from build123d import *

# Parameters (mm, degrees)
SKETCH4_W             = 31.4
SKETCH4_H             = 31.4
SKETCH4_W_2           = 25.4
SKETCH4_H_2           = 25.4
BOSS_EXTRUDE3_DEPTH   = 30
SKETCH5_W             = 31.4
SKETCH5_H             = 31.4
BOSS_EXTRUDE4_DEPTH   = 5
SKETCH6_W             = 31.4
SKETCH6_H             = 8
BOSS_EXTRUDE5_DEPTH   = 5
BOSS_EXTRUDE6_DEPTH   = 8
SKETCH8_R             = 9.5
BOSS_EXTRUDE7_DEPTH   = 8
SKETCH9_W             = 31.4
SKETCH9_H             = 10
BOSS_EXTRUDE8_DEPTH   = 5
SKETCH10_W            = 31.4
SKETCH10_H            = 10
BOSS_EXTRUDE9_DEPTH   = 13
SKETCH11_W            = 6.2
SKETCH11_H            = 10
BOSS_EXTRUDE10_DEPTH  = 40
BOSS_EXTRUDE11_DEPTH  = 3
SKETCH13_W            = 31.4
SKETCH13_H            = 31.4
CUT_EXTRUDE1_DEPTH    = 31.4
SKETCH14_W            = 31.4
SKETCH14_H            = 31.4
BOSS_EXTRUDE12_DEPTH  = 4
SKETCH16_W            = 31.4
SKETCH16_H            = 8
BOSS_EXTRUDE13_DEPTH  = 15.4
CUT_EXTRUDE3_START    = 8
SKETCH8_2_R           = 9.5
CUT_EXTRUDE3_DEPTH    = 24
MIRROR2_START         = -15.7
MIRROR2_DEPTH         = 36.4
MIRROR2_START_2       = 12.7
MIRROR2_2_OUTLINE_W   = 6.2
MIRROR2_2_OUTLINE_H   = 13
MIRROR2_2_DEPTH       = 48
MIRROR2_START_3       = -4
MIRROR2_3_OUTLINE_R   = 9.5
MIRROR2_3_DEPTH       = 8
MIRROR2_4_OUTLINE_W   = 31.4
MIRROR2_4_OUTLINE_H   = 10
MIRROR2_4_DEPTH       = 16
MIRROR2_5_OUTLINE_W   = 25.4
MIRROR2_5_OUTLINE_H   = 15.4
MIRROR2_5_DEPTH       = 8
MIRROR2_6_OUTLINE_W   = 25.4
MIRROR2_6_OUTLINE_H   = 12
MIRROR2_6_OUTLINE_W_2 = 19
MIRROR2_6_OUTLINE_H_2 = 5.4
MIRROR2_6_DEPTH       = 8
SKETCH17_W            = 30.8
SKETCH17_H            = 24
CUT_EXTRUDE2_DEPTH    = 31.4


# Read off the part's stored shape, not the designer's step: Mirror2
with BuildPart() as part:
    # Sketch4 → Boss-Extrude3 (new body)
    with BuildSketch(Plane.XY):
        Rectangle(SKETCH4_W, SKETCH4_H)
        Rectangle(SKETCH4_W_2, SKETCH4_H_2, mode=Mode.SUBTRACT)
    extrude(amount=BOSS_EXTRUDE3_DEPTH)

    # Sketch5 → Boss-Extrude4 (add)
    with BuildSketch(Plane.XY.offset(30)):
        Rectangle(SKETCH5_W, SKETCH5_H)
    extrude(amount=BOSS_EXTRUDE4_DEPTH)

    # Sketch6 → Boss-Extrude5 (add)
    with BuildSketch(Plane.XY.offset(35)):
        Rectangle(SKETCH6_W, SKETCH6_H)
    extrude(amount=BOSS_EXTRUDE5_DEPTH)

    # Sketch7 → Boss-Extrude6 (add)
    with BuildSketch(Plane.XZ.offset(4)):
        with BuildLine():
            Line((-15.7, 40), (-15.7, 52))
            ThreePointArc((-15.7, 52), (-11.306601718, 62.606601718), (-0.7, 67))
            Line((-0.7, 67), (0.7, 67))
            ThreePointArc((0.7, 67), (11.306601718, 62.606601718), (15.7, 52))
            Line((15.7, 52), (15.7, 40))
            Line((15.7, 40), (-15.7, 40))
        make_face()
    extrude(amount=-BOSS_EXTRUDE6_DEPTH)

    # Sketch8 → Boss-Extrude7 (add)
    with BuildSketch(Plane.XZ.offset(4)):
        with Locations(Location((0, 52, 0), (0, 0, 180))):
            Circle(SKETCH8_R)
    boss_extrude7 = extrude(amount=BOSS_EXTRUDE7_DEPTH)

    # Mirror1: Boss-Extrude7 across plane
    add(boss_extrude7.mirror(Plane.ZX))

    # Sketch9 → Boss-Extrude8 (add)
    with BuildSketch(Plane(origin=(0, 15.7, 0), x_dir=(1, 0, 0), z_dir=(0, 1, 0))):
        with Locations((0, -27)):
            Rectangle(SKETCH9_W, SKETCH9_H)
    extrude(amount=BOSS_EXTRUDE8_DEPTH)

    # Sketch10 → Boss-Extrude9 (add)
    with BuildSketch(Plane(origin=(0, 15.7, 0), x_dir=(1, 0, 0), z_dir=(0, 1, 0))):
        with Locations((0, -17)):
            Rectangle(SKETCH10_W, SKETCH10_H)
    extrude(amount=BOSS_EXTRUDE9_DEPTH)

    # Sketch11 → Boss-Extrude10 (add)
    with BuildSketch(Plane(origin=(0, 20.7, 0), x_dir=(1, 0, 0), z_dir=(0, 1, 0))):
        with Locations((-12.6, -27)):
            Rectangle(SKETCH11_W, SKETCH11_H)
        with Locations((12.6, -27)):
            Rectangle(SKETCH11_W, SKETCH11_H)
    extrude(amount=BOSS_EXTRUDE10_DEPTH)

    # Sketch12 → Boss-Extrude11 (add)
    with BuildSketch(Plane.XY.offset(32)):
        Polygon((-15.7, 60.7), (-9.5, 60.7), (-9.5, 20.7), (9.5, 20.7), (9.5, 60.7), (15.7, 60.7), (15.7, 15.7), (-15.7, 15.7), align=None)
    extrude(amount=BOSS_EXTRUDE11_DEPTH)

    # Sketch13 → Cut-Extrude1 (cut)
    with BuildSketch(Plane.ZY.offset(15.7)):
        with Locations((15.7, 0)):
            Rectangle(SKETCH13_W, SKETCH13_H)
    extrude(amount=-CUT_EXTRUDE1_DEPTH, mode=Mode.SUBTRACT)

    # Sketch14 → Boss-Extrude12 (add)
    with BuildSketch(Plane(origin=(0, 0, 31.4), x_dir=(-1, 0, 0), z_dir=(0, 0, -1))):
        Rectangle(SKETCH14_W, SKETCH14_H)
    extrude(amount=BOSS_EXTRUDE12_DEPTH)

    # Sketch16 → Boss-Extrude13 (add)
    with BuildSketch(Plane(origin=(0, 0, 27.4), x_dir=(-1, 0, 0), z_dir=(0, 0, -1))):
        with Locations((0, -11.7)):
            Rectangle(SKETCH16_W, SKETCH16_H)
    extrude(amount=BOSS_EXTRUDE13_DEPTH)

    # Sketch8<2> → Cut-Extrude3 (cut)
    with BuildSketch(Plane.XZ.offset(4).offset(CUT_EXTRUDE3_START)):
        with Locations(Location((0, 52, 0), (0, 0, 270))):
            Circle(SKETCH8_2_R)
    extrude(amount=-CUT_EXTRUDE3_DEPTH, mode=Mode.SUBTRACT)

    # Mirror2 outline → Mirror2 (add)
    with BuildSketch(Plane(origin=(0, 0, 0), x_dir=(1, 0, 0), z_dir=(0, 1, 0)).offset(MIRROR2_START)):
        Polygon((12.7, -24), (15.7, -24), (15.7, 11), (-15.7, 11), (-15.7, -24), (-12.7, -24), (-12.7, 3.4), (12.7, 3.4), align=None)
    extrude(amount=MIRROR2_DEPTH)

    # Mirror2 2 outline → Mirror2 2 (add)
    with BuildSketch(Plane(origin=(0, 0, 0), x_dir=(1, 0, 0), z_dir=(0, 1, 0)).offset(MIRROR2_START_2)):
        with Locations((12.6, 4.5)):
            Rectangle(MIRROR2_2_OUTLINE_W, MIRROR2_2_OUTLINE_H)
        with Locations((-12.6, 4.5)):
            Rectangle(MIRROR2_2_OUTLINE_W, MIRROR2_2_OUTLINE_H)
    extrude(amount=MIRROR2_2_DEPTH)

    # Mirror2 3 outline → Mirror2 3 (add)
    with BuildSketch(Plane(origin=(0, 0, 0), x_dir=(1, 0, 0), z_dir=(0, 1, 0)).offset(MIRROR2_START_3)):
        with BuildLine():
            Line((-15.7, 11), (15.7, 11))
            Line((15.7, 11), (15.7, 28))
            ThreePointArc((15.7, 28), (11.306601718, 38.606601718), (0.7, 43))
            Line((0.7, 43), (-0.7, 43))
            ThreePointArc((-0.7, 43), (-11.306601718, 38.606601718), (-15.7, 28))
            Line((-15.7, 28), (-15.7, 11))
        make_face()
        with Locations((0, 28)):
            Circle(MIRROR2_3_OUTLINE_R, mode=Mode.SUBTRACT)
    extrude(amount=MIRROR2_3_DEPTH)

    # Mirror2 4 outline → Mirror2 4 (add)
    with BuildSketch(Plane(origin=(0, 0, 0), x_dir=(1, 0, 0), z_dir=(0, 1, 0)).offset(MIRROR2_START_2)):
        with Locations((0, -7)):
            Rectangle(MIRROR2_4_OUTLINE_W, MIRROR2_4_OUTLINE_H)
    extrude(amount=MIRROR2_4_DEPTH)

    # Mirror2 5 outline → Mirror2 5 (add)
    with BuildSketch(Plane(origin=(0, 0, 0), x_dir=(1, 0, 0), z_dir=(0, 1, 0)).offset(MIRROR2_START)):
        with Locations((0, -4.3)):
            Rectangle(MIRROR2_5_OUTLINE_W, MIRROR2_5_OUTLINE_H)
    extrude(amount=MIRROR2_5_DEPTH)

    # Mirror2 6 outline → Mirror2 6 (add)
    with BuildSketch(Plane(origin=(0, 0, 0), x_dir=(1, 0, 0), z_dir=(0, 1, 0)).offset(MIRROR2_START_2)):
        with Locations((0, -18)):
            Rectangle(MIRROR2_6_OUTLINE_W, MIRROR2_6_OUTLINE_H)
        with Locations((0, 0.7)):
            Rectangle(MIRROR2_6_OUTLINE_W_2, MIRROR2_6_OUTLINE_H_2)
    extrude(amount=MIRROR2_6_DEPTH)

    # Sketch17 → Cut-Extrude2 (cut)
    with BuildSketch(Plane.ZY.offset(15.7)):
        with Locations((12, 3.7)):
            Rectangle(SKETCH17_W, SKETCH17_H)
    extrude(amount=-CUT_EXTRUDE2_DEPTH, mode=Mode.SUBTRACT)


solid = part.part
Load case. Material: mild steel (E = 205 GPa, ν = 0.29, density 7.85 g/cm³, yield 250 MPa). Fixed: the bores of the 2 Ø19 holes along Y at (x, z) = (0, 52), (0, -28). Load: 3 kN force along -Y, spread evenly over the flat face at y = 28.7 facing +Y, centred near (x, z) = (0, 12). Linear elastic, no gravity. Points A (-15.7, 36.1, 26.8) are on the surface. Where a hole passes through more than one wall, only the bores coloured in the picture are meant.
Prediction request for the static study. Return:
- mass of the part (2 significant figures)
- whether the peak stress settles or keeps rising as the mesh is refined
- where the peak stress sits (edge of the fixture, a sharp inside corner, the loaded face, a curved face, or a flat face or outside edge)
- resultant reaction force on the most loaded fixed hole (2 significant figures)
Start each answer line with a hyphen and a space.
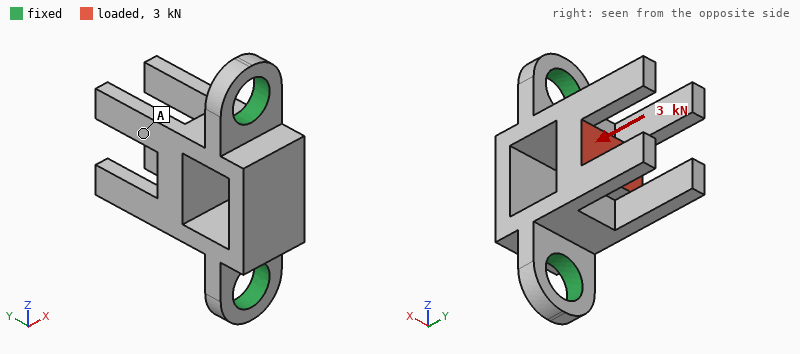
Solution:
- 450 g
- keeps rising
- edge of the fixture
- 1.6 kN
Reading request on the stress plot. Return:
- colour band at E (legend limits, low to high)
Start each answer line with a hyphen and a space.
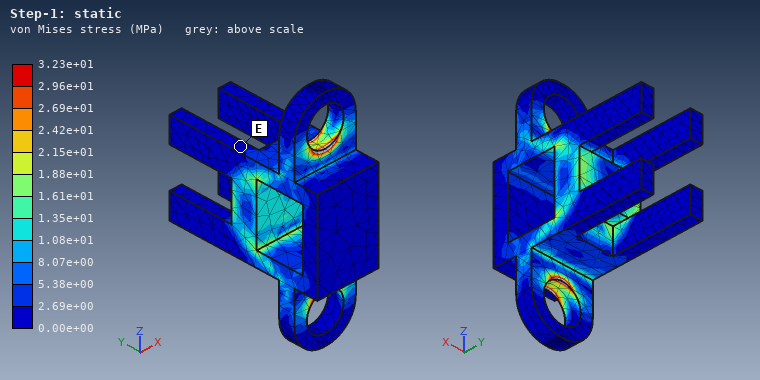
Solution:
- 0.00e+00 to 2.69e+00 MPa
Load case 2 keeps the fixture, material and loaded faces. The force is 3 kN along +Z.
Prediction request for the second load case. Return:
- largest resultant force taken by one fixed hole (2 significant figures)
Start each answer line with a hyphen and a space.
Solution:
- 2.1 kN
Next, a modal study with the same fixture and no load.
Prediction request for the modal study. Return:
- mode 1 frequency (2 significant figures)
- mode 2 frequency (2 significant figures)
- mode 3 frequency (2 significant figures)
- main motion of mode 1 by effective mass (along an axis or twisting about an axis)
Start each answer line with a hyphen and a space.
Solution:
- 2400 Hz
- 3200 Hz
- 3300 Hz
- along X
